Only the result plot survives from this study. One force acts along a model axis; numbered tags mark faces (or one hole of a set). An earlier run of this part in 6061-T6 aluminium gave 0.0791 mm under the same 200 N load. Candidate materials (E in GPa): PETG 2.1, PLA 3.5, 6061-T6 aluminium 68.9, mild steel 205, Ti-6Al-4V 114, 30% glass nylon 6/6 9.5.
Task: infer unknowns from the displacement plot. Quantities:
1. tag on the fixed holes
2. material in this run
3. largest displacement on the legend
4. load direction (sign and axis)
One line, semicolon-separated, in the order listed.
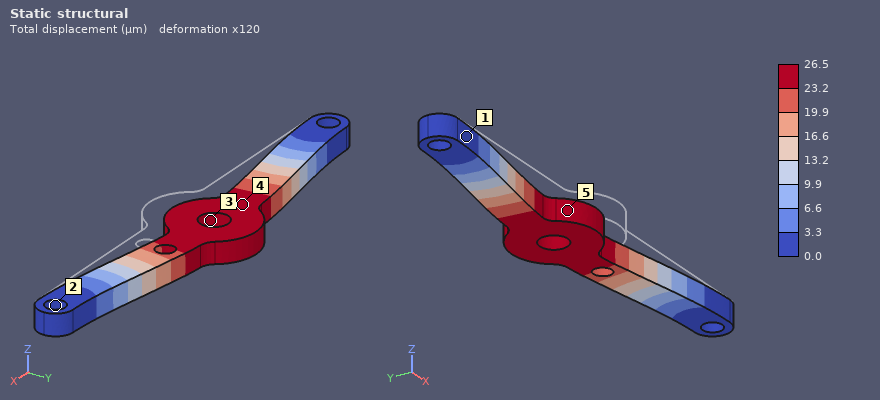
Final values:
2; mild steel; 26.5 µm; +Y
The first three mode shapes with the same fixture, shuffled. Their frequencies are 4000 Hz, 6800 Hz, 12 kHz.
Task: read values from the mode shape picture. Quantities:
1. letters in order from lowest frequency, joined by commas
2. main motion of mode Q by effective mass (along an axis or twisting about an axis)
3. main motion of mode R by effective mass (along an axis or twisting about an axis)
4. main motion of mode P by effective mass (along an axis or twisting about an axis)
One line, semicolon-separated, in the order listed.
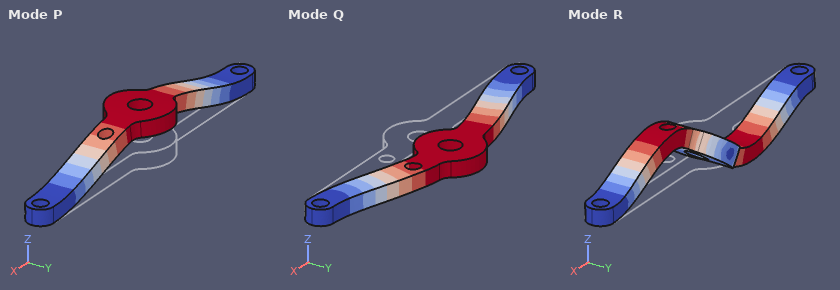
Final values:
P, Q, R; along Y; twisting about Y; along Z
